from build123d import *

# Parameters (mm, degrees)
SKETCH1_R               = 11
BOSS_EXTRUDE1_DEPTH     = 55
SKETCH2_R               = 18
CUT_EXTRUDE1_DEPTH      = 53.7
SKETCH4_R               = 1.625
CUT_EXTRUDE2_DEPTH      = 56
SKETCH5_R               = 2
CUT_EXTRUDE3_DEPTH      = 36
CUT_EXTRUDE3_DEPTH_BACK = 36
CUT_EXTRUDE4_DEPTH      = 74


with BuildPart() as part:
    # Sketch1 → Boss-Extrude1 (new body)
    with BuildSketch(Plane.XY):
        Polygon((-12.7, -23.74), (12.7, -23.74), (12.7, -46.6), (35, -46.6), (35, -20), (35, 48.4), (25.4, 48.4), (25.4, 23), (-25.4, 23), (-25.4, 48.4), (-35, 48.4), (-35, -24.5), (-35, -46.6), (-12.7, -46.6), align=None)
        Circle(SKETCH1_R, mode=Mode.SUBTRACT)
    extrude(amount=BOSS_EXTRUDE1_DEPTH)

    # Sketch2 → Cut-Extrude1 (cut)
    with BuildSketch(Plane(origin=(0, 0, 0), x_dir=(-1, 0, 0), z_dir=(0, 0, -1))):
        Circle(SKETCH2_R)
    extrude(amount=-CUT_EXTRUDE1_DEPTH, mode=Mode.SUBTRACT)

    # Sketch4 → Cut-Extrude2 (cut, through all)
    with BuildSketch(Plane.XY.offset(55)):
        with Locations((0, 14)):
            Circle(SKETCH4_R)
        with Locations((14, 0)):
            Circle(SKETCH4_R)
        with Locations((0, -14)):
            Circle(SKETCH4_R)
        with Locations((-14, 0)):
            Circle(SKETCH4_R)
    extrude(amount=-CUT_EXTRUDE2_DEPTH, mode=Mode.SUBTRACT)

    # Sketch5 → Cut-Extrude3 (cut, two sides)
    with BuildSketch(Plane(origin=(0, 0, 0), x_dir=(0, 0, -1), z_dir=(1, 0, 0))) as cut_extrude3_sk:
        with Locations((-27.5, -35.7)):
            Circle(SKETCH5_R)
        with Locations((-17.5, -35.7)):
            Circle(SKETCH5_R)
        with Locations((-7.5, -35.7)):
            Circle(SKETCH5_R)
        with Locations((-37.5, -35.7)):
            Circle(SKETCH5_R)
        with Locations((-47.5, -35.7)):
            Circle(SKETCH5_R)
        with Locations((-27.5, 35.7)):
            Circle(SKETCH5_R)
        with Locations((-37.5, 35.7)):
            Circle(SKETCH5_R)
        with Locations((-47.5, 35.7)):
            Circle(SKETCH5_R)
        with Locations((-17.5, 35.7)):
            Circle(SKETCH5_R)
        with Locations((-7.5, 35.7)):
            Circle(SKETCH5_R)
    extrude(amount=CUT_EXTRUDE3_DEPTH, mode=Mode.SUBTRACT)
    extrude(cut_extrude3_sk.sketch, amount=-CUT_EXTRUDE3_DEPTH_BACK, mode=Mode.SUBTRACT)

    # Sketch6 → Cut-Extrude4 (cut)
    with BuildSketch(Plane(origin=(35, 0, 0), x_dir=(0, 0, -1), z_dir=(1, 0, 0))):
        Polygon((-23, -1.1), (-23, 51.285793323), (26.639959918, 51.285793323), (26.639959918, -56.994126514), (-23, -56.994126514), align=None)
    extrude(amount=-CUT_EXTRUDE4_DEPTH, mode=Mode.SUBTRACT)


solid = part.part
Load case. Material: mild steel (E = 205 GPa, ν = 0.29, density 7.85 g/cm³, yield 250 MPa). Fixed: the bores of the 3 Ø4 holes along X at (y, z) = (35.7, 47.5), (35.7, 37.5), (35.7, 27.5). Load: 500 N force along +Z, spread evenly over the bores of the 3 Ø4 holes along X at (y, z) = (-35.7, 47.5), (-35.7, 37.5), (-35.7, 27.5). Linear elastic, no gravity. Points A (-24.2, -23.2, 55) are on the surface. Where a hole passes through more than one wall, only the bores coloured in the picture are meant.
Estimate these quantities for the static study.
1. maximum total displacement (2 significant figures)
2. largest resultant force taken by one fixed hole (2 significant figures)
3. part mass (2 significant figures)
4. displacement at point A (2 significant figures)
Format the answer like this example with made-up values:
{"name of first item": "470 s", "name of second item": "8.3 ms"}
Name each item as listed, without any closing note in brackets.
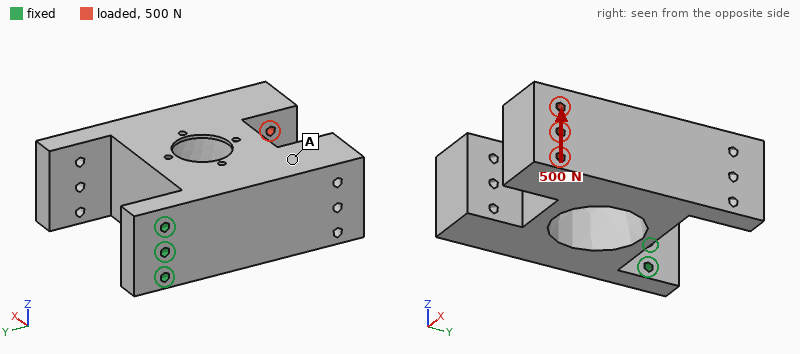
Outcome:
{"maximum total displacement": "46 µm", "largest resultant force taken by one fixed hole": "2.0 kN", "part mass": "930 g", "displacement at point A": "12 µm"}
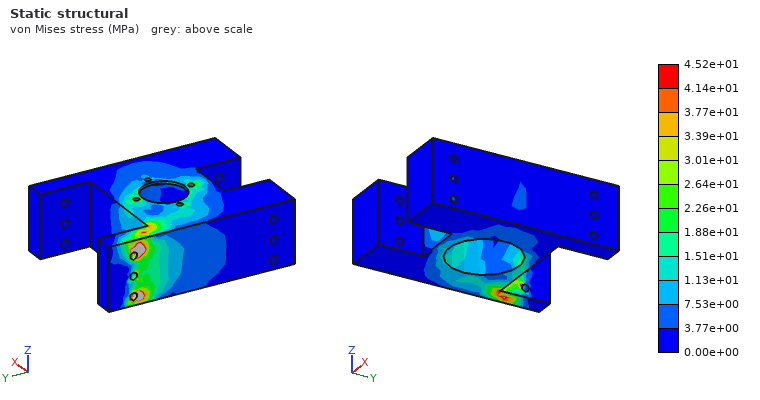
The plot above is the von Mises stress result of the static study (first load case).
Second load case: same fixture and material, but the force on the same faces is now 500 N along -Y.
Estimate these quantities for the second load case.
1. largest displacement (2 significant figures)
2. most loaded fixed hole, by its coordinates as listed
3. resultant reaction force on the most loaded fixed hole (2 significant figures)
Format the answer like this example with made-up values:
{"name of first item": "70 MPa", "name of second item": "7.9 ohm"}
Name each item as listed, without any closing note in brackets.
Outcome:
{"largest displacement": "97 µm", "most loaded fixed hole, by its coordinates as listed": "(35.7, 37.5)", "resultant reaction force on the most loaded fixed hole": "220 N"}
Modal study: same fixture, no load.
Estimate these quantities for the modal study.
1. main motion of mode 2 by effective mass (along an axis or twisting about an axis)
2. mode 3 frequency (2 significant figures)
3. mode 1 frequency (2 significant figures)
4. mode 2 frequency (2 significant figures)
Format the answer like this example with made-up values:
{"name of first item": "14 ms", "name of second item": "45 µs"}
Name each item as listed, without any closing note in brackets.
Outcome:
{"main motion of mode 2 by effective mass": "along Z", "mode 3 frequency": "2100 Hz", "mode 1 frequency": "490 Hz", "mode 2 frequency": "990 Hz"}
